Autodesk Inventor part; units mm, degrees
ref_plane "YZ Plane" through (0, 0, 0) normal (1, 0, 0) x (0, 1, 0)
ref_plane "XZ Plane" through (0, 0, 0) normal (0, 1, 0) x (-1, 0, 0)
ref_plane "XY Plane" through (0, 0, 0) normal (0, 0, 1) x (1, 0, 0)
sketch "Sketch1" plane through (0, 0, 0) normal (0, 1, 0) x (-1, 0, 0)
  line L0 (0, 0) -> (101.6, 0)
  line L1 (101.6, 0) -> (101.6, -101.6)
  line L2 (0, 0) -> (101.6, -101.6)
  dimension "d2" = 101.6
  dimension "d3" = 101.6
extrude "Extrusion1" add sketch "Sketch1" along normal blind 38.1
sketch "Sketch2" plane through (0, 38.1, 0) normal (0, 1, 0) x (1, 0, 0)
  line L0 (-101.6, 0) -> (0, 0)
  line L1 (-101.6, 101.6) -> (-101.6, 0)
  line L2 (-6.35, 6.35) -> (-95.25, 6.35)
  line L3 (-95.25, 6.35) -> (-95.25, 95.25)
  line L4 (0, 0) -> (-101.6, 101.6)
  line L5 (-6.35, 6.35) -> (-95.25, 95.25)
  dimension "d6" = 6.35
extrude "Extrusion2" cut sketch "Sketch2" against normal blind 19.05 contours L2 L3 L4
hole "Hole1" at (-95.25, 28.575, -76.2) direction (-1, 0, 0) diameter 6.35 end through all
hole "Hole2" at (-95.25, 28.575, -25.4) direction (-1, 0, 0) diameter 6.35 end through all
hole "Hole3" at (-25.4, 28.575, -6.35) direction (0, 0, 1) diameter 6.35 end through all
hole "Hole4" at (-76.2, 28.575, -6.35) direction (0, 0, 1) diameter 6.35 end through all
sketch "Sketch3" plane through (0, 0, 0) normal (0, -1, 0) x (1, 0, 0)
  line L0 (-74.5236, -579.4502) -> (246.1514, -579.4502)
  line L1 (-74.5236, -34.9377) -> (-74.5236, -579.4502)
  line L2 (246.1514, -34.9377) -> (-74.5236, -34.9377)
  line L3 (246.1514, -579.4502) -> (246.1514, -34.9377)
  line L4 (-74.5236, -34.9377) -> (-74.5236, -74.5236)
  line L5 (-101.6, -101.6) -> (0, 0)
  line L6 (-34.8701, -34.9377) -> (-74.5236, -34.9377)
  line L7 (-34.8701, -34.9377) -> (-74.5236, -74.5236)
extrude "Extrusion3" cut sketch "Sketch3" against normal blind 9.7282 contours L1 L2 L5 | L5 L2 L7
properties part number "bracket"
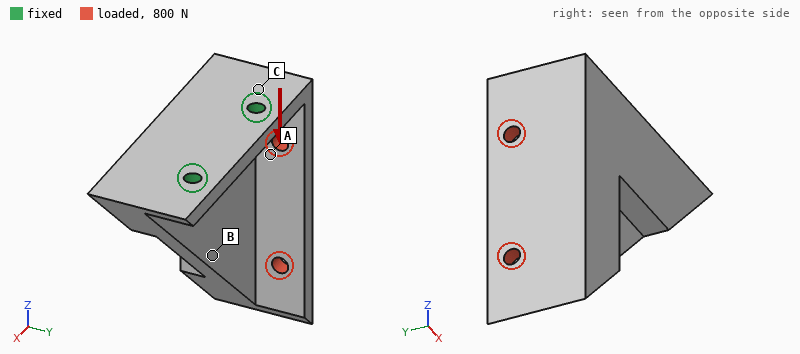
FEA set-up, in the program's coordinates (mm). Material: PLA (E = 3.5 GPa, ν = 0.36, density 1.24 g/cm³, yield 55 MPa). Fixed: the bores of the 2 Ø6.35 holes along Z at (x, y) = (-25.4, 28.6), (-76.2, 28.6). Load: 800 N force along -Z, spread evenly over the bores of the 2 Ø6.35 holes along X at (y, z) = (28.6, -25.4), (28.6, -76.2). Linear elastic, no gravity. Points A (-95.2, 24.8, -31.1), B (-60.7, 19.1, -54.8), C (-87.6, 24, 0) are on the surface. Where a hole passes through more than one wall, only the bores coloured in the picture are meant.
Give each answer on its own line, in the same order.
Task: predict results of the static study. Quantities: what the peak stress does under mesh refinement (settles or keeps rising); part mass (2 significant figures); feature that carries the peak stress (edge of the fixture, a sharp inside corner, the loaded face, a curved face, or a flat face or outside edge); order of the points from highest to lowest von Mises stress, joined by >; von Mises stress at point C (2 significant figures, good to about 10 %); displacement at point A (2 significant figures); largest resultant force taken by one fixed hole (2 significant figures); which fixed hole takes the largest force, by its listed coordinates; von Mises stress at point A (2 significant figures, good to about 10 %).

keeps rising
140 g
edge of the fixture
C > A > B
12 MPa
0.34 mm
1.1 kN
(-76.2, 28.6)
5.3 MPa
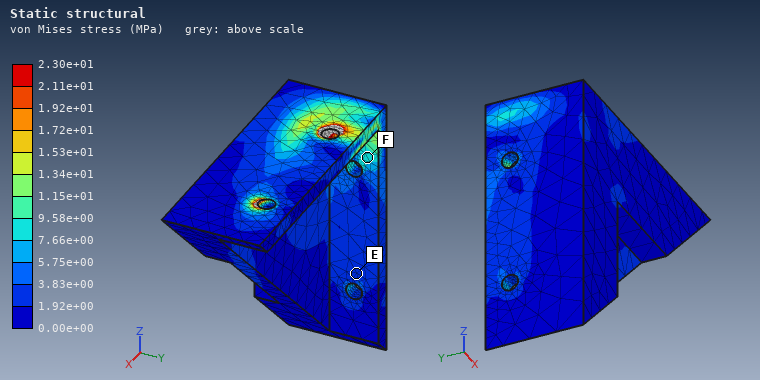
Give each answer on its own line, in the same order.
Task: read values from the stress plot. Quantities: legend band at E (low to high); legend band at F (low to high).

1.92e+00 to 3.83e+00 MPa
7.66e+00 to 9.58e+00 MPa
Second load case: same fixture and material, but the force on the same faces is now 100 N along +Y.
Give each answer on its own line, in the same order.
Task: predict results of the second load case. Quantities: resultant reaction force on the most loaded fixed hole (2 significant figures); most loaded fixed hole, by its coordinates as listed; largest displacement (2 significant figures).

140 N
(-76.2, 28.6)
1.1 mm
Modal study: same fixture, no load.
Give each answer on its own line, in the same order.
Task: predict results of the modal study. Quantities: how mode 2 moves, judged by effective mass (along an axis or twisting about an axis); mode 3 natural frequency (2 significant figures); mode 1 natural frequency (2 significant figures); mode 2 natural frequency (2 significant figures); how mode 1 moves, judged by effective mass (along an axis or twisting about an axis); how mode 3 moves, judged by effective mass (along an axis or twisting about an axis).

along X
1300 Hz
230 Hz
740 Hz
along Y
along Z
